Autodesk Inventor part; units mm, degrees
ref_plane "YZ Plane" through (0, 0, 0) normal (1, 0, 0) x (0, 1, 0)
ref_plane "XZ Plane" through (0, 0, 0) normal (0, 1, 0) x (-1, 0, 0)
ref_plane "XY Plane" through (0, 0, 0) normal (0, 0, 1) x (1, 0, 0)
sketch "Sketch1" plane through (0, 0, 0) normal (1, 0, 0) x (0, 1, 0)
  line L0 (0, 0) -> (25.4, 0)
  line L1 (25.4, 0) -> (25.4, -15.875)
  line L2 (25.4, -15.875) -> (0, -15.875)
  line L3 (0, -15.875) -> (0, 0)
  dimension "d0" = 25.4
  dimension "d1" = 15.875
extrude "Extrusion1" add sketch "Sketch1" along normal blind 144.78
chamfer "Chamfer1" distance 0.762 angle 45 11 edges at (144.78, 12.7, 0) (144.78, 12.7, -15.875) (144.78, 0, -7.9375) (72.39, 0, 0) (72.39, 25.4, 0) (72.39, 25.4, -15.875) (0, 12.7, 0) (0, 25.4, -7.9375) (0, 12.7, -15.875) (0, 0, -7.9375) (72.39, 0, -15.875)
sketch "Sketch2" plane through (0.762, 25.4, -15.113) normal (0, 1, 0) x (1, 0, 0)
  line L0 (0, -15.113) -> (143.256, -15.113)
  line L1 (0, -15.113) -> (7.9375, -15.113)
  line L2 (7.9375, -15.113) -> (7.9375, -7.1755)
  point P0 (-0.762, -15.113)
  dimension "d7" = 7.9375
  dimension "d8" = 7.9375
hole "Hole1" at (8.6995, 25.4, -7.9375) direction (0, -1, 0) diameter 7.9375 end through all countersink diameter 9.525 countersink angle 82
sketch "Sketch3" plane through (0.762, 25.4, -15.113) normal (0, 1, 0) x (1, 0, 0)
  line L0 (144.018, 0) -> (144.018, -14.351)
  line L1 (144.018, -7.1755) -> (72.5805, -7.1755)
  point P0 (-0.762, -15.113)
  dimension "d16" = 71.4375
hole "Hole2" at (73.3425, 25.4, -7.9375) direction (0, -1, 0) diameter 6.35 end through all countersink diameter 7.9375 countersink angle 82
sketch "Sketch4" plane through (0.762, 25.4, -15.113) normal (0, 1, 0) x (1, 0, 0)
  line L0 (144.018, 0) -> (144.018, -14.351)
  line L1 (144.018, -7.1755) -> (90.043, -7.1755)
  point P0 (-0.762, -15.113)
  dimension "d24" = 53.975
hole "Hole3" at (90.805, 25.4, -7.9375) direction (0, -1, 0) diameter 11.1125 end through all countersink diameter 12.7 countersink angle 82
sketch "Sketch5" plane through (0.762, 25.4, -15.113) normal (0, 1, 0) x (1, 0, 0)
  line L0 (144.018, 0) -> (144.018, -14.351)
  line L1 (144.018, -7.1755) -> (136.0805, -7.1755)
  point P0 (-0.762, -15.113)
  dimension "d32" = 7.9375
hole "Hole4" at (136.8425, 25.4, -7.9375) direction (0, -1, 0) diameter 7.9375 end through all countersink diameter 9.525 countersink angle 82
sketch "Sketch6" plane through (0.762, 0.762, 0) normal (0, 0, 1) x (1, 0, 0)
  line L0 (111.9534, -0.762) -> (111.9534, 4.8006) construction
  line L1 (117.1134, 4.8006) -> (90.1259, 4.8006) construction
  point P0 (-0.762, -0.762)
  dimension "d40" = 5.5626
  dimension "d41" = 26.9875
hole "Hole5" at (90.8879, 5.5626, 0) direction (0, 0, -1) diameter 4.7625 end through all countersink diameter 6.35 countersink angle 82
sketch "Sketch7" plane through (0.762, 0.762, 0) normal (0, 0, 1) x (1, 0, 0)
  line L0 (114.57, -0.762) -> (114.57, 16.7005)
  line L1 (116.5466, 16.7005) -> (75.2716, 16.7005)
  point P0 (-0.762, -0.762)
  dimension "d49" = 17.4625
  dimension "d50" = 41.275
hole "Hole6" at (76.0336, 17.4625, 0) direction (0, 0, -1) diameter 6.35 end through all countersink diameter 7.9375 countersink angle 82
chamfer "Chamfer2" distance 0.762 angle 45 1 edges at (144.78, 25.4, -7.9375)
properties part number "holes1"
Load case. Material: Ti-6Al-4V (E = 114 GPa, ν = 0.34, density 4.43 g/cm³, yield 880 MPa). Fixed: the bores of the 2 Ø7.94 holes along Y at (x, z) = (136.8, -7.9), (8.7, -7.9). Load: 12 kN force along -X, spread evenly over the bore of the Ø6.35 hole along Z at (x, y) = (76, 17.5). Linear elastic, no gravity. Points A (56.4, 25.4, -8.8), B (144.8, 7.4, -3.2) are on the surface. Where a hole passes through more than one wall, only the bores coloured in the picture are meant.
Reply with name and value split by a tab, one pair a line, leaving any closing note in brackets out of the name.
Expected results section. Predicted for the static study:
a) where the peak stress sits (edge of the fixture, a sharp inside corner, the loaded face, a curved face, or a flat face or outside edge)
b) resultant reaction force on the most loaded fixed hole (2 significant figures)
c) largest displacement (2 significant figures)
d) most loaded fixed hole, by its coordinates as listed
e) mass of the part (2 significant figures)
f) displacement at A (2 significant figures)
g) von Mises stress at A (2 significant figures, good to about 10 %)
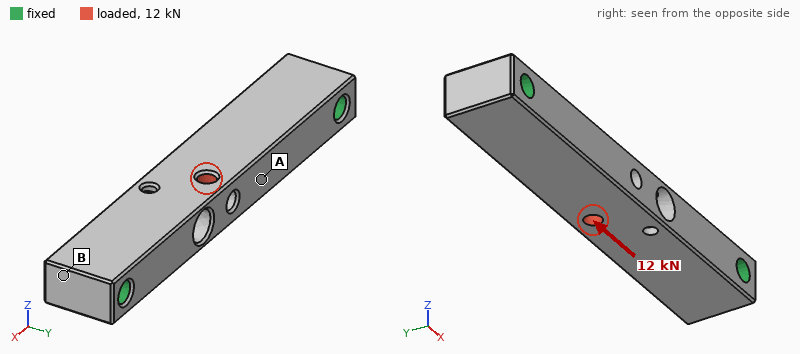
where the peak stress sits	the loaded face
resultant reaction force on the most loaded fixed hole	6.8 kN
largest displacement	16 µm
most loaded fixed hole, by its coordinates as listed	(8.7, -7.9)
mass of the part	230 g
displacement at A	7.8 µm
von Mises stress at A	27 MPa
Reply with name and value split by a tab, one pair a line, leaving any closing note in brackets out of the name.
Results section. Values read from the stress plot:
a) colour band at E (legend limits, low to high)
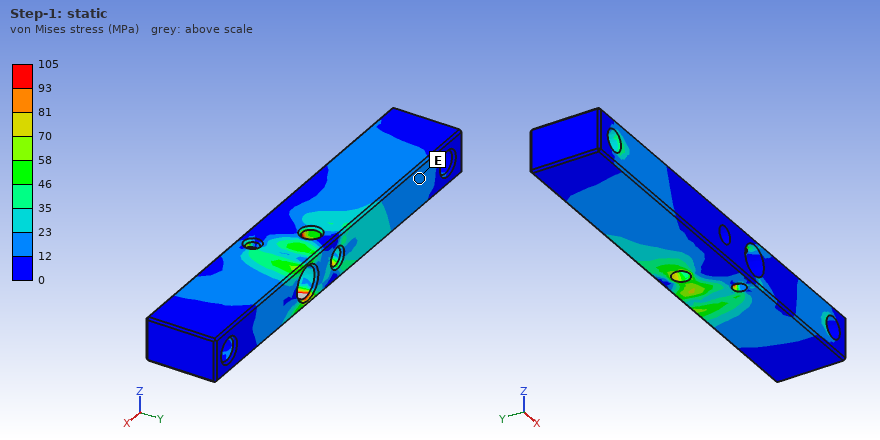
colour band at E	12 to 23 MPa
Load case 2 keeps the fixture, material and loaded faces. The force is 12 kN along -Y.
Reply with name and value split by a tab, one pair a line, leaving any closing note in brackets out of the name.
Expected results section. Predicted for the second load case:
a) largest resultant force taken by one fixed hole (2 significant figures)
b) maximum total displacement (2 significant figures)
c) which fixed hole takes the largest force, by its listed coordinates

largest resultant force taken by one fixed hole	6.6 kN
maximum total displacement	0.10 mm
which fixed hole takes the largest force, by its listed coordinates	(136.8, -7.9)
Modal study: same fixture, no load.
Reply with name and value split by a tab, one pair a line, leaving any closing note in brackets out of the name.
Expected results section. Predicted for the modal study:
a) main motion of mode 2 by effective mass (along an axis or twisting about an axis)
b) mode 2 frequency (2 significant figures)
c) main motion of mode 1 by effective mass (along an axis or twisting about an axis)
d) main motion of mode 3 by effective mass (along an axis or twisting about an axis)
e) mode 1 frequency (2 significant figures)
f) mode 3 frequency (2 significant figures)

main motion of mode 2 by effective mass	along Y
mode 2 frequency	6800 Hz
main motion of mode 1 by effective mass	along Z
main motion of mode 3 by effective mass	twisting about X
mode 1 frequency	4600 Hz
mode 3 frequency	11 kHz
